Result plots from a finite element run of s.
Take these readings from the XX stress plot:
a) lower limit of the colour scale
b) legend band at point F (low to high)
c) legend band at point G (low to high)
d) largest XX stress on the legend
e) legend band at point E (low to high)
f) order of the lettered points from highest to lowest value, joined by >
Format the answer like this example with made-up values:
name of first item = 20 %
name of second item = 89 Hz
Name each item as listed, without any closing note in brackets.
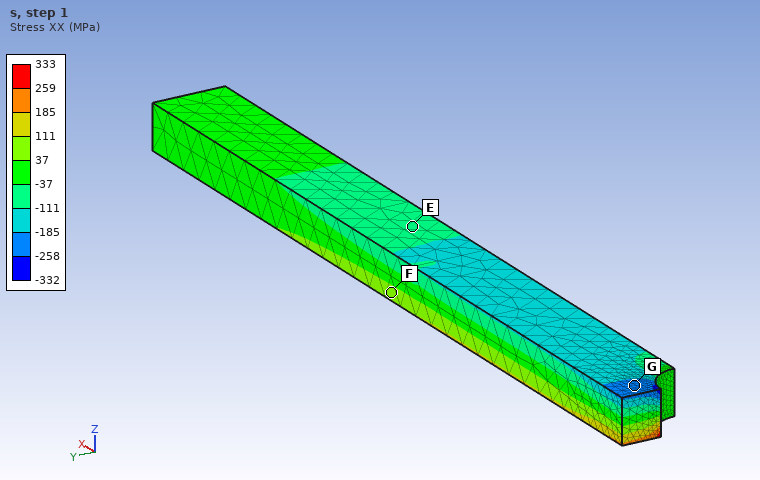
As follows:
lower limit of the colour scale = -332 MPa
legend band at point F = 37 to 111 MPa
legend band at point G = -258 to -185 MPa
largest XX stress on the legend = 333 MPa
legend band at point E = -111 to -37 MPa
order of the lettered points from highest to lowest value, joined by > = F > E > G
